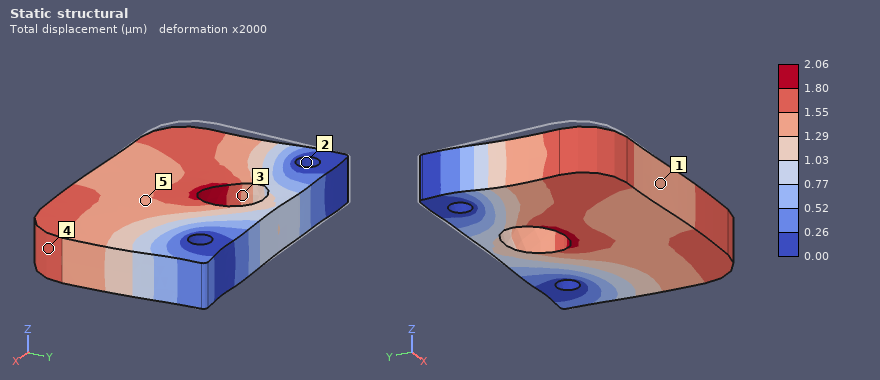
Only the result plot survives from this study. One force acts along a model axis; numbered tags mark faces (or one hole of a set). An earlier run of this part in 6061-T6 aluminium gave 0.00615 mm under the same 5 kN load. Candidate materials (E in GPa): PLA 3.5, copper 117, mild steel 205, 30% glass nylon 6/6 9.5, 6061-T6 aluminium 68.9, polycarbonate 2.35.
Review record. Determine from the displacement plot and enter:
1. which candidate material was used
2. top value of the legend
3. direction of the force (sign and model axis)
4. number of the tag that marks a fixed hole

mild steel
2.06 µm
+X
2
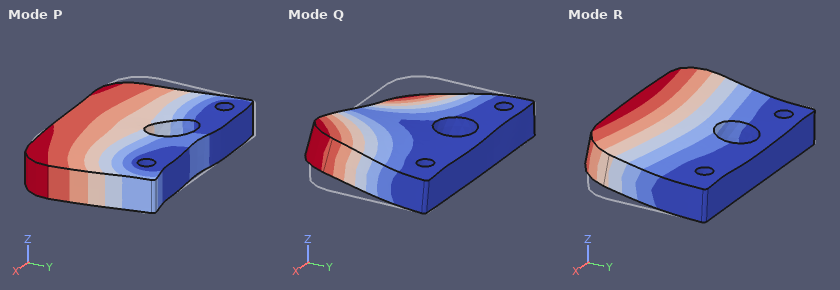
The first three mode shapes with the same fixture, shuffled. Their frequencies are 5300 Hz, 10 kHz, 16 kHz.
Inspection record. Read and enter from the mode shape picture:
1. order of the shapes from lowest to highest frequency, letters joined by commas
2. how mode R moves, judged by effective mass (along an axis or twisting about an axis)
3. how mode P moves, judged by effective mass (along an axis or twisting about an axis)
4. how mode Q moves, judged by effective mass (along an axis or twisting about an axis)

R, Q, P
along Z
along X
twisting about Y
